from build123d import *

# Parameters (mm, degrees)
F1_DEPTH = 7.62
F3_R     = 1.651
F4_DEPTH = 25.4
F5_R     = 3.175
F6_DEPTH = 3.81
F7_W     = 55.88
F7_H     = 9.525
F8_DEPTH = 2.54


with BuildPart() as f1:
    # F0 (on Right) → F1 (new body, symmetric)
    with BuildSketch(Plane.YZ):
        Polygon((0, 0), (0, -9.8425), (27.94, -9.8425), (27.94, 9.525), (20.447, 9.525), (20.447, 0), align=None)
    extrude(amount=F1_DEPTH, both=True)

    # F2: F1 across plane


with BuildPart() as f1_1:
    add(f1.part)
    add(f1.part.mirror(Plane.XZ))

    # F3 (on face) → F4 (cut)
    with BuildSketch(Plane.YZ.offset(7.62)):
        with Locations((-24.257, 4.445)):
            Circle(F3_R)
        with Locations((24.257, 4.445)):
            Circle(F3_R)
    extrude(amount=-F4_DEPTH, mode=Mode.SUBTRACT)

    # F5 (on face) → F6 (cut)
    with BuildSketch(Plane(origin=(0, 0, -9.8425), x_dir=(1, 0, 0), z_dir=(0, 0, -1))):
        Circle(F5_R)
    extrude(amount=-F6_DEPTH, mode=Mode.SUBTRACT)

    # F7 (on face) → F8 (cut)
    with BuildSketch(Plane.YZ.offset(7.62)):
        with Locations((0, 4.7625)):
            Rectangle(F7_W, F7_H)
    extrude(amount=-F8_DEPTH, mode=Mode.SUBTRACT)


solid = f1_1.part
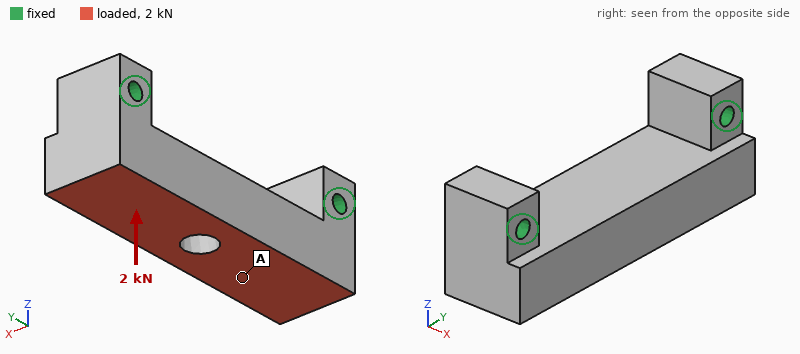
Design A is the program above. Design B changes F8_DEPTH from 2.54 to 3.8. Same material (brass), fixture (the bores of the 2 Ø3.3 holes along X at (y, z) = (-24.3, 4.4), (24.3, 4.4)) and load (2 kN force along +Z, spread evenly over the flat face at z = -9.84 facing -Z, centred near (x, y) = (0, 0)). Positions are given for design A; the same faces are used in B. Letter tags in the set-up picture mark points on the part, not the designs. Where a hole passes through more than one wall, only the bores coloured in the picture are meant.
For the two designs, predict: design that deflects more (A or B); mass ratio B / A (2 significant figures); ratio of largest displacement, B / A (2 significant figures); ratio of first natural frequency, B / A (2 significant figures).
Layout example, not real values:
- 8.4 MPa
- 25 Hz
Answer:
- B
- 0.98
- 1.1
- 0.92
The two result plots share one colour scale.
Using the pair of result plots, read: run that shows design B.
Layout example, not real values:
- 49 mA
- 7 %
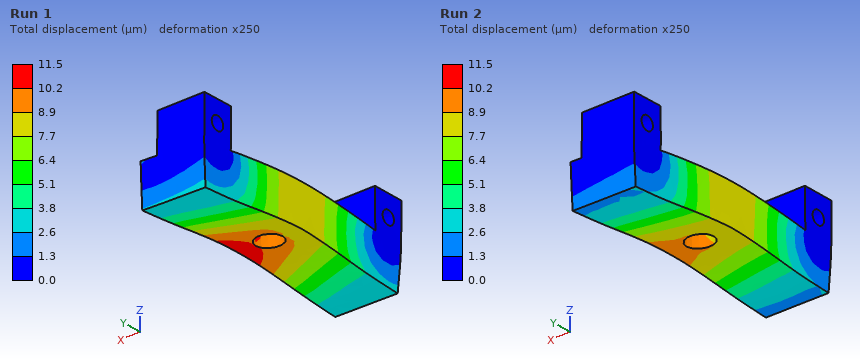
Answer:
- Run 1
